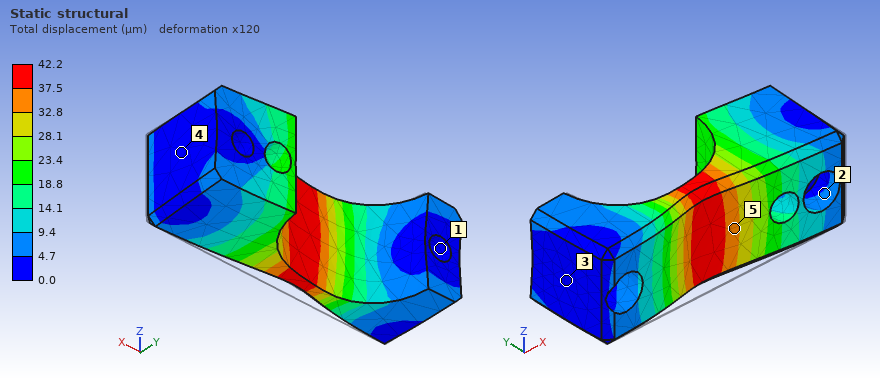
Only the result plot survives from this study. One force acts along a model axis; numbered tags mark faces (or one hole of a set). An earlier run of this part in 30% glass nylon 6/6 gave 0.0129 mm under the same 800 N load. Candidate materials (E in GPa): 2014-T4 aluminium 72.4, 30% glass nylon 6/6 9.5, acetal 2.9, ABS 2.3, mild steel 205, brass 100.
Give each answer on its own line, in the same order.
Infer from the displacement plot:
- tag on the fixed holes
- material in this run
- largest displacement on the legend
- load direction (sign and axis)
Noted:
1
acetal
42.2 µm
+Y
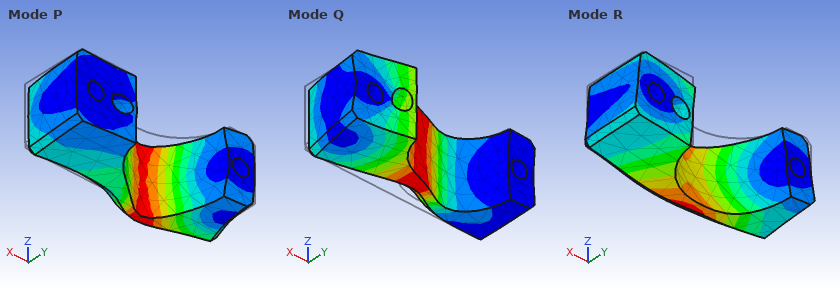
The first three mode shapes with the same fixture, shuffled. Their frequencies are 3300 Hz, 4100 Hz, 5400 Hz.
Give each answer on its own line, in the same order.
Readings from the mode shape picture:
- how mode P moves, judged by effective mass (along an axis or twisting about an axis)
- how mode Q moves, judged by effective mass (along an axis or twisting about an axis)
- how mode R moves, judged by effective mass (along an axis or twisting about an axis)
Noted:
along X
along Y
along Z
